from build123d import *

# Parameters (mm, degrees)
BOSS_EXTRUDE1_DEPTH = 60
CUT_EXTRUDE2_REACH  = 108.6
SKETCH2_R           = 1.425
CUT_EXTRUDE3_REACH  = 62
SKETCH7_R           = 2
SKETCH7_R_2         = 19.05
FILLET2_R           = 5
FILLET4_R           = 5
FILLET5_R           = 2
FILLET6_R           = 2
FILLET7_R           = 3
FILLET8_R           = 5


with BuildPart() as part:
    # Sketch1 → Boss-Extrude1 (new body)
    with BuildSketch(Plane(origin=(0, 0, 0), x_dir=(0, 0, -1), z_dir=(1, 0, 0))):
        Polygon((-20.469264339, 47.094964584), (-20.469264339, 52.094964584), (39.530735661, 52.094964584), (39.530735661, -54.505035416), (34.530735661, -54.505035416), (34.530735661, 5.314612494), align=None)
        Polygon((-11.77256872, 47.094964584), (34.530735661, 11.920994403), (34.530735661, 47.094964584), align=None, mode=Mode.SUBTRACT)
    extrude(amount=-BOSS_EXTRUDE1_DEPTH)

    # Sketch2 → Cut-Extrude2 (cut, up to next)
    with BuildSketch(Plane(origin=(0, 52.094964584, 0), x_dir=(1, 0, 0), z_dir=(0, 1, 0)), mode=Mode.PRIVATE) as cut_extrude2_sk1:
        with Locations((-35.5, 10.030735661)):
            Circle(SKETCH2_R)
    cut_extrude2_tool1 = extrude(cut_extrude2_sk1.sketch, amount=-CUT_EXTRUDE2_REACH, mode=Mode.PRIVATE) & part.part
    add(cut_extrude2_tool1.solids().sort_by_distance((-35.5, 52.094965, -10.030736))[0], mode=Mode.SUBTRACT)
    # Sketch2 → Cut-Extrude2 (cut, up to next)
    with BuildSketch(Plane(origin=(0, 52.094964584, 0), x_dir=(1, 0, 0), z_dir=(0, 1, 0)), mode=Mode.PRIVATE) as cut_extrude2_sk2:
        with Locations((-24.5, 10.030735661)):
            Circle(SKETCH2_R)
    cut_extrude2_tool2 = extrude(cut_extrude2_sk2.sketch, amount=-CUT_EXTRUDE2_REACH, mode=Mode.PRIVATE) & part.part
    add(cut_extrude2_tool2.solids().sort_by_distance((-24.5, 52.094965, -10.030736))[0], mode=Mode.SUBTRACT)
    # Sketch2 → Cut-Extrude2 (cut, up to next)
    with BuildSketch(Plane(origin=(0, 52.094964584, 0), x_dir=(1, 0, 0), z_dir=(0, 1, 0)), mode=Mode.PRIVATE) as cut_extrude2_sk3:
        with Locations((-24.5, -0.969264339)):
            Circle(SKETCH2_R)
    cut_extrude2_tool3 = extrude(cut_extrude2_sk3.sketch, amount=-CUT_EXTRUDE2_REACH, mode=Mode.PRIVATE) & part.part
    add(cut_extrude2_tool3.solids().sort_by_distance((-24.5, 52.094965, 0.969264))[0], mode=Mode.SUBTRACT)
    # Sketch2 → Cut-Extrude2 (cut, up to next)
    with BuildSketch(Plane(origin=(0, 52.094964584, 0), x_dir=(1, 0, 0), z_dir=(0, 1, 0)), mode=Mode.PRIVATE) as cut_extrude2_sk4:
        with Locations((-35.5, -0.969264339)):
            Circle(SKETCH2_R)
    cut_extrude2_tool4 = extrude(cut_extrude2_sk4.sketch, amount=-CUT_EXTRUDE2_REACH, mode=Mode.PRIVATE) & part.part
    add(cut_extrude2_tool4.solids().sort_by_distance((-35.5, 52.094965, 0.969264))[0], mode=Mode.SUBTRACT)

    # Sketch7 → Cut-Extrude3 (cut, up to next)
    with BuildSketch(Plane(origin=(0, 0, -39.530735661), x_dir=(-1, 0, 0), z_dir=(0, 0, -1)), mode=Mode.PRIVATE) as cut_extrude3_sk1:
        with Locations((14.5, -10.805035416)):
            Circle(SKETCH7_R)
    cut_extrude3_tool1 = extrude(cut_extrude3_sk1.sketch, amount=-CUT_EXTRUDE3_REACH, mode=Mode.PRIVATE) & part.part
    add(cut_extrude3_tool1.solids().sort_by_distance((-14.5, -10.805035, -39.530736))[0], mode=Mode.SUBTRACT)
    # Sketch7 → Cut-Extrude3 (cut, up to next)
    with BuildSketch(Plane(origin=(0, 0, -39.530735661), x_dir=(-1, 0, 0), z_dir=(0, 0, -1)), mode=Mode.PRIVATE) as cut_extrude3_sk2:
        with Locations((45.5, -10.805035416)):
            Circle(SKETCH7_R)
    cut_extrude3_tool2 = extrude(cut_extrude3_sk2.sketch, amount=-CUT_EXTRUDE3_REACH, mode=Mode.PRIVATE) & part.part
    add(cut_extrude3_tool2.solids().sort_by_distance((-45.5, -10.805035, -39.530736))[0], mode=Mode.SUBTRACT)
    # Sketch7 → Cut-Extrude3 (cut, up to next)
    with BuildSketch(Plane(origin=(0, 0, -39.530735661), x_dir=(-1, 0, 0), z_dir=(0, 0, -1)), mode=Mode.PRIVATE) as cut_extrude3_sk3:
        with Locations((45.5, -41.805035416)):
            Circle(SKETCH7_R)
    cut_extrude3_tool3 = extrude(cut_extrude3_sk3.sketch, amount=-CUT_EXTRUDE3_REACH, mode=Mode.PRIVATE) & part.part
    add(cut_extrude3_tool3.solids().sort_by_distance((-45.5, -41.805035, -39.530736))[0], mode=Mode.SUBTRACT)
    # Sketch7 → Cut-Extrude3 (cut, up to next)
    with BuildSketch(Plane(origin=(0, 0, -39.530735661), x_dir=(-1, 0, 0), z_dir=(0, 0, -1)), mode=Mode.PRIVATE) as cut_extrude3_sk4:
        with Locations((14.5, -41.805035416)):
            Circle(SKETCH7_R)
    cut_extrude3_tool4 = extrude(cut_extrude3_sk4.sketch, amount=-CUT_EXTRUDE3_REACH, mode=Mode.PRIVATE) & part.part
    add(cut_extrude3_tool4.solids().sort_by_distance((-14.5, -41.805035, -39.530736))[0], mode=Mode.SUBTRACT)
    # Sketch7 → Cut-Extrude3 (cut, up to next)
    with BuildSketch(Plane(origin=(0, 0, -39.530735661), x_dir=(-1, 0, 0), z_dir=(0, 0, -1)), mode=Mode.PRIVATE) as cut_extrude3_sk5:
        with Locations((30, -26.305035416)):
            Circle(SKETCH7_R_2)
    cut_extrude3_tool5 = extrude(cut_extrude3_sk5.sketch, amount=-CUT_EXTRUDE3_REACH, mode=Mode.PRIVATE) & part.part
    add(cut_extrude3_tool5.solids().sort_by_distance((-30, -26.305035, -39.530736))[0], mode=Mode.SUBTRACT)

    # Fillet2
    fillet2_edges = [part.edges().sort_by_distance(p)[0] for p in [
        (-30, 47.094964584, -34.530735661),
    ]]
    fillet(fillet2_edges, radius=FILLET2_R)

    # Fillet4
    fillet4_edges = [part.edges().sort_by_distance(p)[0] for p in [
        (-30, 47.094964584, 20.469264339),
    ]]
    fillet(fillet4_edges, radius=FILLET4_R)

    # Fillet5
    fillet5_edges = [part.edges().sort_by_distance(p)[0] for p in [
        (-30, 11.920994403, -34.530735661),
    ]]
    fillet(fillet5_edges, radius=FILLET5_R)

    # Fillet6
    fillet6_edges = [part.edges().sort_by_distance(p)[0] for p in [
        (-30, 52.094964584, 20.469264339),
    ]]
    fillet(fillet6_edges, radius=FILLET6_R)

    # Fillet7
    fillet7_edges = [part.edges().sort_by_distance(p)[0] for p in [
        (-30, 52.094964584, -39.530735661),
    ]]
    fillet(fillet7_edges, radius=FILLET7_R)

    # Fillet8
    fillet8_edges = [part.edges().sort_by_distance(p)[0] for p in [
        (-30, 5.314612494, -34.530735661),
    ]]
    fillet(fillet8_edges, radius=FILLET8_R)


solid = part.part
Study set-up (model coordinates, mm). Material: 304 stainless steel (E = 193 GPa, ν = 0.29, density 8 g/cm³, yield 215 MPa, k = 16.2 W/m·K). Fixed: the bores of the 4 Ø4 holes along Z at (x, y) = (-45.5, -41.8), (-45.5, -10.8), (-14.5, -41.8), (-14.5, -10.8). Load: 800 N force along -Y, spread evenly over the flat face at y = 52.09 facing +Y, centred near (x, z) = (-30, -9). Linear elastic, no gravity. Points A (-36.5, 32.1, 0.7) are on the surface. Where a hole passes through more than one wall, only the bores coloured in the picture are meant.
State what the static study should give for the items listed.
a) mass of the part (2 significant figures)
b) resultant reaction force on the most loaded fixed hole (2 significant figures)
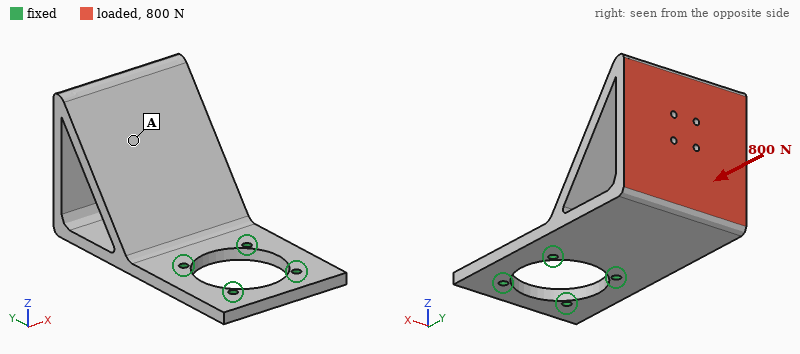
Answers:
500 g
390 N
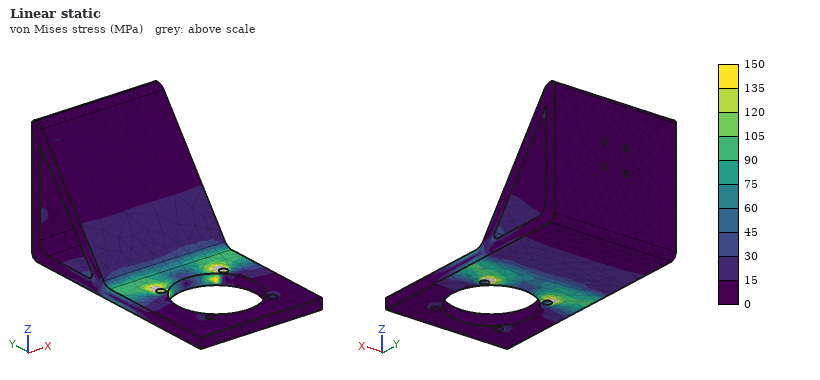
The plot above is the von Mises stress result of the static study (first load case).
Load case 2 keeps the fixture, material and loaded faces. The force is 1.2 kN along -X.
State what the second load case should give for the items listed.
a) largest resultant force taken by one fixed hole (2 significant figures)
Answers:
2.0 kN
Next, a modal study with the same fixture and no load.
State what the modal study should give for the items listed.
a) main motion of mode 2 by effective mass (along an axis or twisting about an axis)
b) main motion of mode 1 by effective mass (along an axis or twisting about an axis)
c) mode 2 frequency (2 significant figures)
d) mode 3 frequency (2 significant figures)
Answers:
along X
along Z
1400 Hz
3200 Hz
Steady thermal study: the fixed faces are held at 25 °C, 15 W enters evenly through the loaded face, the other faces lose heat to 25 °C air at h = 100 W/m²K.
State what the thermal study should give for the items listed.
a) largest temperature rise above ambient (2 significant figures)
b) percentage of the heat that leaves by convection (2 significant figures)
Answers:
23 K
98 %
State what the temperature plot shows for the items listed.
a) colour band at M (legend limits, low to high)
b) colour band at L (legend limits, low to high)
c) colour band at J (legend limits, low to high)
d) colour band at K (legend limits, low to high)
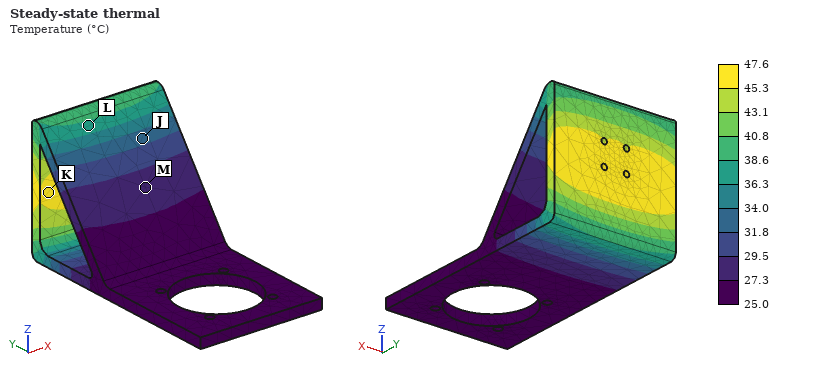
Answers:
27.3 to 29.5 °C
36.3 to 38.6 °C
31.8 to 34.0 °C
45.3 to 47.6 °C
